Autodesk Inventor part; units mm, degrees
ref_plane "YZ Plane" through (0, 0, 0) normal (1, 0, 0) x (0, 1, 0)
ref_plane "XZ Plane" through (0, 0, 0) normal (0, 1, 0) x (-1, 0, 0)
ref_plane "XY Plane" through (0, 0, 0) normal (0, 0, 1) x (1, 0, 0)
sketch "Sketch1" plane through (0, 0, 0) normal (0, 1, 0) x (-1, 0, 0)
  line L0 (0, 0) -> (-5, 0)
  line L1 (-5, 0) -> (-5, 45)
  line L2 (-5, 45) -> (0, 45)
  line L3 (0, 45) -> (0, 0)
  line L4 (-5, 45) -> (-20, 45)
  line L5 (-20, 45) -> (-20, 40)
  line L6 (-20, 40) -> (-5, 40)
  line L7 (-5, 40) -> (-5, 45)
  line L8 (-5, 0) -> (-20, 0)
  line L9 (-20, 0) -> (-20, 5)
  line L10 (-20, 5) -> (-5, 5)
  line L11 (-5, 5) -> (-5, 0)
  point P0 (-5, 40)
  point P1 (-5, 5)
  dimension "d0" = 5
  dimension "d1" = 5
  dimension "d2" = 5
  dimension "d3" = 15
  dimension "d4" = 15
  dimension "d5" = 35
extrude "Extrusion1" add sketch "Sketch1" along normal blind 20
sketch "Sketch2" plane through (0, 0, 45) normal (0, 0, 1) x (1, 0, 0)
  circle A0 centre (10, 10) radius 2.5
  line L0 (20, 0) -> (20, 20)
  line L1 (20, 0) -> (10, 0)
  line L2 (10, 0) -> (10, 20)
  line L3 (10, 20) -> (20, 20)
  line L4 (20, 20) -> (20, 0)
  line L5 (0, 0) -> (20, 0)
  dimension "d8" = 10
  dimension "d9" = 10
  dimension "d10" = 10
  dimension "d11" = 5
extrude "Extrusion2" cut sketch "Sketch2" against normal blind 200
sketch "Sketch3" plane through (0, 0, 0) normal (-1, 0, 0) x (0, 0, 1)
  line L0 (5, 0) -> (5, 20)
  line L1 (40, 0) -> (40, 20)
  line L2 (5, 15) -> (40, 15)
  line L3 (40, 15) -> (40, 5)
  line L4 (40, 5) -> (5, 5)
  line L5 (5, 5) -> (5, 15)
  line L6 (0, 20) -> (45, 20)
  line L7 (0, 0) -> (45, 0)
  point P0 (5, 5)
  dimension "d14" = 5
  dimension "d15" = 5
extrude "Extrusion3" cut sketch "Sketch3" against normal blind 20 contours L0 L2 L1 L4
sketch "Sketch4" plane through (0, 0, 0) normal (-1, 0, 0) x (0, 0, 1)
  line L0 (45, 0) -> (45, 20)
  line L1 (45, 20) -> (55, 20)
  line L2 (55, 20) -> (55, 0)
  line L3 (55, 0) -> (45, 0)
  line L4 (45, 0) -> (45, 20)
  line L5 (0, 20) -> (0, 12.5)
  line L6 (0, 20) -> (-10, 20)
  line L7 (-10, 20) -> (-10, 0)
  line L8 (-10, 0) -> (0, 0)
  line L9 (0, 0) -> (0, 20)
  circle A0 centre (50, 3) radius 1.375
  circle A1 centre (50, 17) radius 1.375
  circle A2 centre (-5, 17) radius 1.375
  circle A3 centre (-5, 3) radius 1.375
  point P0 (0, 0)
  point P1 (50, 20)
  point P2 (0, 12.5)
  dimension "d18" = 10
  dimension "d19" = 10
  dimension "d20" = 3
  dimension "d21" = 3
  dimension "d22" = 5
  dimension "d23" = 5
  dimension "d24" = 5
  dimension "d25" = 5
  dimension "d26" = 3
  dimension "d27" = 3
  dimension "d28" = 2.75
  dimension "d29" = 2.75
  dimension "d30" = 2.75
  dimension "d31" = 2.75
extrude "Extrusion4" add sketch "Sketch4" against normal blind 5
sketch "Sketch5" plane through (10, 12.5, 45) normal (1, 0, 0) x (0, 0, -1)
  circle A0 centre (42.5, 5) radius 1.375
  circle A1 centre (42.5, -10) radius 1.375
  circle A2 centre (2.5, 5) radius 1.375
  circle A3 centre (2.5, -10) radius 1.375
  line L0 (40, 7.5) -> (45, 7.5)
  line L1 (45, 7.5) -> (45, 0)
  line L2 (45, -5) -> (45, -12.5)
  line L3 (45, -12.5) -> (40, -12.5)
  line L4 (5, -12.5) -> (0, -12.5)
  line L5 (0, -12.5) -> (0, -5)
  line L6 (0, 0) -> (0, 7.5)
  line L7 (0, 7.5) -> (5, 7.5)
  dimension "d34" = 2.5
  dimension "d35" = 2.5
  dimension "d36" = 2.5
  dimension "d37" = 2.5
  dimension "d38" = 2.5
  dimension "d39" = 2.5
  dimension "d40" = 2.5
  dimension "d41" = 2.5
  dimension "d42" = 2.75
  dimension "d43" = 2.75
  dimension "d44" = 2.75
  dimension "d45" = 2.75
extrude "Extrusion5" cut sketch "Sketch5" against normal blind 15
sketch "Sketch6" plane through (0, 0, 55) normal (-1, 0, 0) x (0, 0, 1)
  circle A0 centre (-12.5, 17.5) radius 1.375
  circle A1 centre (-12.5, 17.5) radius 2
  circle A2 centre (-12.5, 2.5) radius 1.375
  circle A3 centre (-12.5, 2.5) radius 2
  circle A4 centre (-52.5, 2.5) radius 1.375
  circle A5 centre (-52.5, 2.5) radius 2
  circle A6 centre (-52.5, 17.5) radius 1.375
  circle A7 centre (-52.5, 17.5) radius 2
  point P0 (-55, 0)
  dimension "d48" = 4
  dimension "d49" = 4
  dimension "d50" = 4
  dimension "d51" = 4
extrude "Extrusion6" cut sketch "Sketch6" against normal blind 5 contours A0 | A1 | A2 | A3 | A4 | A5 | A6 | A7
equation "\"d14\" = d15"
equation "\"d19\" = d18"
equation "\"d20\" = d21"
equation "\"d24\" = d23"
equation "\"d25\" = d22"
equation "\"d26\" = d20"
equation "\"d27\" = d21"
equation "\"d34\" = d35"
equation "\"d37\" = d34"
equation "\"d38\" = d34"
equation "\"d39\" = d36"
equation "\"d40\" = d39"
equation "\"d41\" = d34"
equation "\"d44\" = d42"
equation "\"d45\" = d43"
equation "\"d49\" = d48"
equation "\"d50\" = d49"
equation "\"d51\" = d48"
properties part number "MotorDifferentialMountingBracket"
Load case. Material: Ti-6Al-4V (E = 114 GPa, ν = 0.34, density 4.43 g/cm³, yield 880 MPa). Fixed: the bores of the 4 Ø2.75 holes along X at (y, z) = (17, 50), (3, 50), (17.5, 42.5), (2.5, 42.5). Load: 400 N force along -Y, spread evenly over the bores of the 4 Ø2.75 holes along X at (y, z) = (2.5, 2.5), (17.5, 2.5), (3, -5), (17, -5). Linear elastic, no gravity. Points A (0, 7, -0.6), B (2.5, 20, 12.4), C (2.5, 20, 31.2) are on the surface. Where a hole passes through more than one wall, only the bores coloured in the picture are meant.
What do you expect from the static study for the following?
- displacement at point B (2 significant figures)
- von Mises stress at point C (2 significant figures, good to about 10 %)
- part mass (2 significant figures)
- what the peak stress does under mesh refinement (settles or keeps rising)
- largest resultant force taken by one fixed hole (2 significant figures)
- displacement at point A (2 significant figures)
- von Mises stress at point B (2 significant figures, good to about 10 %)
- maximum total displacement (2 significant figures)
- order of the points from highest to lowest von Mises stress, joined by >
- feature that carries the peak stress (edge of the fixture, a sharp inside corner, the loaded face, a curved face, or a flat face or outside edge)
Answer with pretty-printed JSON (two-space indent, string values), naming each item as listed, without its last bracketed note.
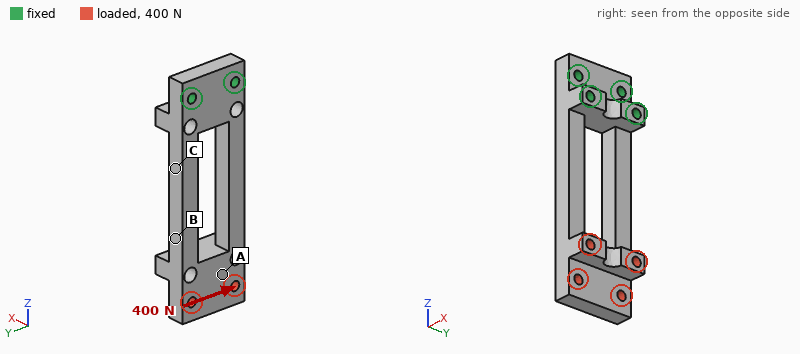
{
  "displacement at point B": "0.22 mm",
  "von Mises stress at point C": "120 MPa",
  "part mass": "23 g",
  "what the peak stress does under mesh refinement": "keeps rising",
  "largest resultant force taken by one fixed hole": "510 N",
  "displacement at point A": "0.25 mm",
  "von Mises stress at point B": "71 MPa",
  "maximum total displacement": "0.30 mm",
  "order of the points from highest to lowest von Mises stress, joined by >": "C > B > A",
  "feature that carries the peak stress": "a sharp inside corner"
}
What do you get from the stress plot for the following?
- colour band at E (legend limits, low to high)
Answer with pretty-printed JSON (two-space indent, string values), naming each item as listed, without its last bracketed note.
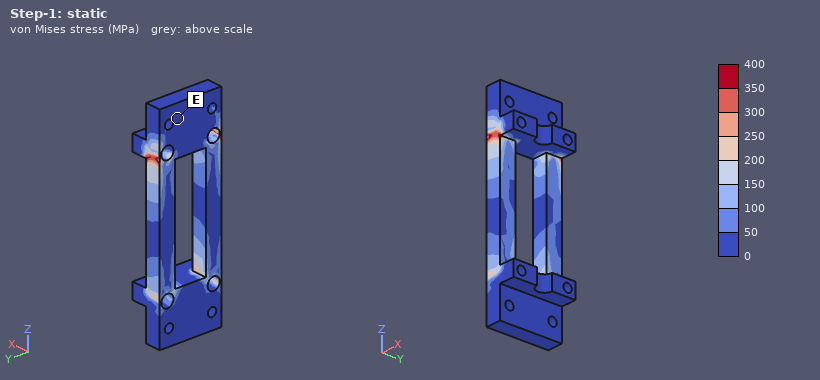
{
  "colour band at E": "0 to 50 MPa"
}
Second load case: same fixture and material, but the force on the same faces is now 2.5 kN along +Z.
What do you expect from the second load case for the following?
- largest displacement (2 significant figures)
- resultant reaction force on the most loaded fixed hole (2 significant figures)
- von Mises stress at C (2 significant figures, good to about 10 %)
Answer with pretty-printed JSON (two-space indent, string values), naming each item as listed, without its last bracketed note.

{
  "largest displacement": "0.68 mm",
  "resultant reaction force on the most loaded fixed hole": "940 N",
  "von Mises stress at C": "45 MPa"
}
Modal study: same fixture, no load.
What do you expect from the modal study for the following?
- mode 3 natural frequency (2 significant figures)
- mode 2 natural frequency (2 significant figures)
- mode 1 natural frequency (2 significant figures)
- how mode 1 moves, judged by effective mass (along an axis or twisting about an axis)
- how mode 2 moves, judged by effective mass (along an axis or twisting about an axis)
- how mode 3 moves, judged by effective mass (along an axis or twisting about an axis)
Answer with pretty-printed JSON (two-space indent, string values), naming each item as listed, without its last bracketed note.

{
  "mode 3 natural frequency": "4100 Hz",
  "mode 2 natural frequency": "1900 Hz",
  "mode 1 natural frequency": "1000 Hz",
  "how mode 1 moves, judged by effective mass": "along X",
  "how mode 2 moves, judged by effective mass": "along Y",
  "how mode 3 moves, judged by effective mass": "twisting about Z"
}
